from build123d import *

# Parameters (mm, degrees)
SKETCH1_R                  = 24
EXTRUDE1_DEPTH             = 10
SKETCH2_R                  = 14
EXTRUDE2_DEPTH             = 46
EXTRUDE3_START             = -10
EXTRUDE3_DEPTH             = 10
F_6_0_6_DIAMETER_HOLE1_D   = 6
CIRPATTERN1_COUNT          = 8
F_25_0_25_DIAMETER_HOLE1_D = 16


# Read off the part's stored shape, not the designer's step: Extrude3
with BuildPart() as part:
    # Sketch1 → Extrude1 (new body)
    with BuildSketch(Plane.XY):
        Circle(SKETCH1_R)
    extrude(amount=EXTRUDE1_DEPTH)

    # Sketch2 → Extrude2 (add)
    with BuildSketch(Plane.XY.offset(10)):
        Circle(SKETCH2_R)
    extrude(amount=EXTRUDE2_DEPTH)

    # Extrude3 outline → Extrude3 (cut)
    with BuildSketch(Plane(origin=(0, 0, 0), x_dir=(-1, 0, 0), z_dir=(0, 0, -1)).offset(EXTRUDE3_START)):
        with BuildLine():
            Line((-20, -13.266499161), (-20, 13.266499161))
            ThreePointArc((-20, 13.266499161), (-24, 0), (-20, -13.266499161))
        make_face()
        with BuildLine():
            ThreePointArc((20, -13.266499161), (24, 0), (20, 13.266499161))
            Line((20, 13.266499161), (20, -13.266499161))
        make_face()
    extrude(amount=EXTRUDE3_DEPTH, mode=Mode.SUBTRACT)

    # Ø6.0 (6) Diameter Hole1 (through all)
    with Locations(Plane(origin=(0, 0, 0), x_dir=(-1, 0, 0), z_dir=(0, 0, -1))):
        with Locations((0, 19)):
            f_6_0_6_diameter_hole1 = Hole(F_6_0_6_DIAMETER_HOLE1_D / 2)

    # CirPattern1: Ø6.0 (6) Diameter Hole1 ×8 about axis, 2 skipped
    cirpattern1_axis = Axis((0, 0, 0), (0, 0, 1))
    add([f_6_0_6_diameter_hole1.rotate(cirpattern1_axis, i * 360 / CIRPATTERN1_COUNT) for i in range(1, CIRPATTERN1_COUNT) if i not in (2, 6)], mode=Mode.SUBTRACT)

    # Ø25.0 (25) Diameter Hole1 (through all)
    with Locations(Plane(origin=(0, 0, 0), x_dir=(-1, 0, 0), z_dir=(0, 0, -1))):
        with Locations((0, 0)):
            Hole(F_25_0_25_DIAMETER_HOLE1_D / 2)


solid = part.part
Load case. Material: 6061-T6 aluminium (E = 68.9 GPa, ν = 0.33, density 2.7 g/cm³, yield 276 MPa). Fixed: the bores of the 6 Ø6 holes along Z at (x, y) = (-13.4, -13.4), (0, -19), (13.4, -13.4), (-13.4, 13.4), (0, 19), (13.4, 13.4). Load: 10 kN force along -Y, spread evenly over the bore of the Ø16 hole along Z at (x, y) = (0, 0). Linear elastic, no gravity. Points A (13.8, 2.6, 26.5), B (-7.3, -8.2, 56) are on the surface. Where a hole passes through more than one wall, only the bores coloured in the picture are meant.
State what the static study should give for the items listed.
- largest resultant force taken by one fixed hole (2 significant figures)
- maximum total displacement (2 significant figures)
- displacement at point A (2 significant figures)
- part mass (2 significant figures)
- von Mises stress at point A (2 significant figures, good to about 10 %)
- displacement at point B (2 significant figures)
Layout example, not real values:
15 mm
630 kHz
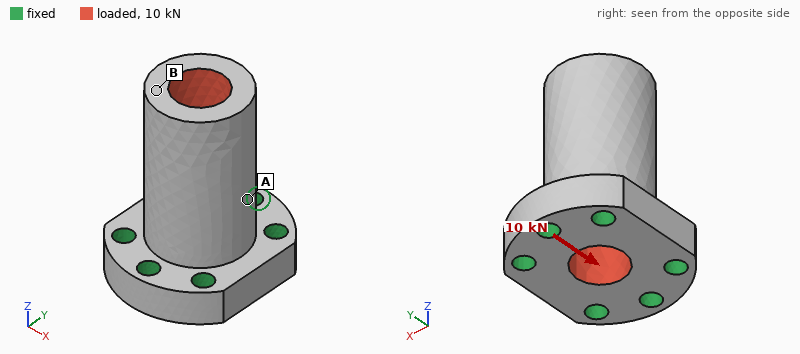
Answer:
4.2 kN
0.12 mm
0.037 mm
86 g
34 MPa
0.11 mm
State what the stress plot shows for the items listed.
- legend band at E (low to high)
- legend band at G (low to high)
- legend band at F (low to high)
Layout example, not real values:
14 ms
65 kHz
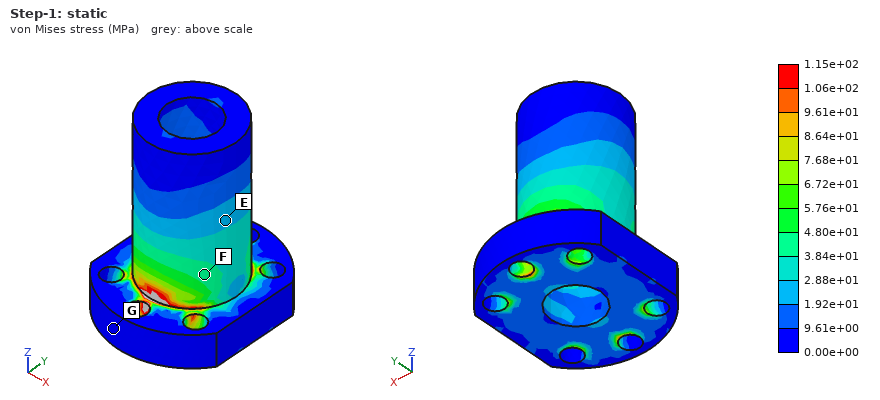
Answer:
1.92e+01 to 2.88e+01 MPa
0.00e+00 to 9.61e+00 MPa
3.84e+01 to 4.80e+01 MPa
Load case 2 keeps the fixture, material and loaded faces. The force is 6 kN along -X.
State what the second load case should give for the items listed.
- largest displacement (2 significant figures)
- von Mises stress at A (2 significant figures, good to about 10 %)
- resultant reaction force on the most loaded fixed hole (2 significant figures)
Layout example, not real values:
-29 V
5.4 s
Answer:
80 µm
23 MPa
3.0 kN
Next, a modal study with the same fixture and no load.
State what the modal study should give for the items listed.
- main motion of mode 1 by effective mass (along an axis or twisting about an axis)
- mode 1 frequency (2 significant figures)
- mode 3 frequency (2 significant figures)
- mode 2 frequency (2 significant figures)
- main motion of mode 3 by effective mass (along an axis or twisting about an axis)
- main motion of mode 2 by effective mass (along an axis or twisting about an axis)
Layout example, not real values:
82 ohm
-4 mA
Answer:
along X
6600 Hz
16 kHz
7100 Hz
twisting about Z
along Y
